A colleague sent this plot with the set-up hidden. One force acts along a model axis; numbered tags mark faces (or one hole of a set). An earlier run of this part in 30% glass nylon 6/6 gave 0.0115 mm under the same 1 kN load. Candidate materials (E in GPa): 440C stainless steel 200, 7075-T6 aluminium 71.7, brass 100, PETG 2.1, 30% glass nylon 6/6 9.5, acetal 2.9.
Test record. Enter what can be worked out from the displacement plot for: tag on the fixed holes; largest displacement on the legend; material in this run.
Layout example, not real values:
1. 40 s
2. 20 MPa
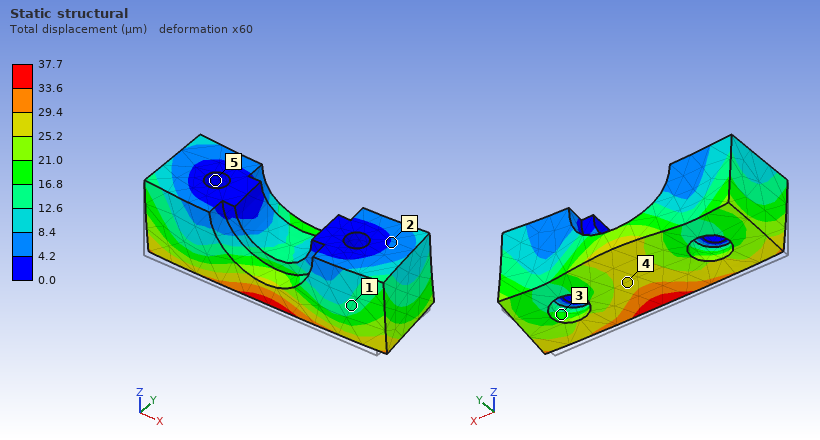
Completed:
1. 5
2. 37.7 µm
3. acetal
